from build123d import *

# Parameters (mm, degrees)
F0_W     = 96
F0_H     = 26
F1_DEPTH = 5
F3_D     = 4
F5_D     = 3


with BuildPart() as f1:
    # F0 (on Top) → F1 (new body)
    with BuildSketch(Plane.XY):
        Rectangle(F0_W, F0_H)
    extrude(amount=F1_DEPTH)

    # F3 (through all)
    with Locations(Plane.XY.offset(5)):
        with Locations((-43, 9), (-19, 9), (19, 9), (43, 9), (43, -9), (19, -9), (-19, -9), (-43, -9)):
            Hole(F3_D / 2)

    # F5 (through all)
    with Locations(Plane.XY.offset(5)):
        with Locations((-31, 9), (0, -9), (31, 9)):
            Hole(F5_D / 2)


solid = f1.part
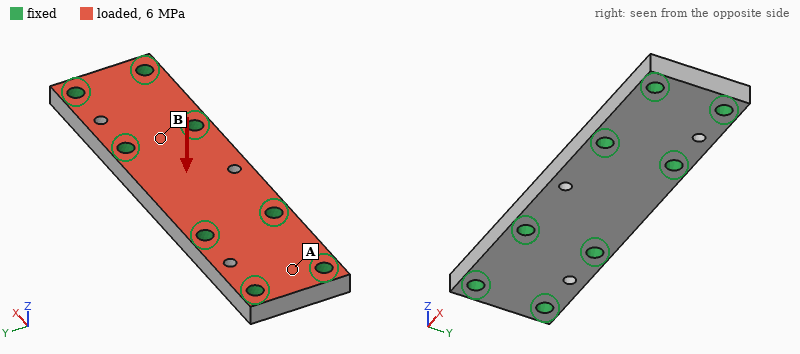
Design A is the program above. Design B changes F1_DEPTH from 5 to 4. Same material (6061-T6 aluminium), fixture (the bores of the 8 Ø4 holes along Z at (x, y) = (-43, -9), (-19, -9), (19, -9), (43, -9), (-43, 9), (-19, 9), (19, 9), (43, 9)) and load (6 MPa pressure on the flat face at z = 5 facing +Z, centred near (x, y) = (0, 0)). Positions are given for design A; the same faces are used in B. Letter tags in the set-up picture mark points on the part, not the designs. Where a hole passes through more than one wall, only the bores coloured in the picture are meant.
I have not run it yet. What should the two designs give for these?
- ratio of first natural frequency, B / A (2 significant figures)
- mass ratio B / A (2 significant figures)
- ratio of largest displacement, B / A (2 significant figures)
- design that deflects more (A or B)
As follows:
0.84
0.80
1.8
B
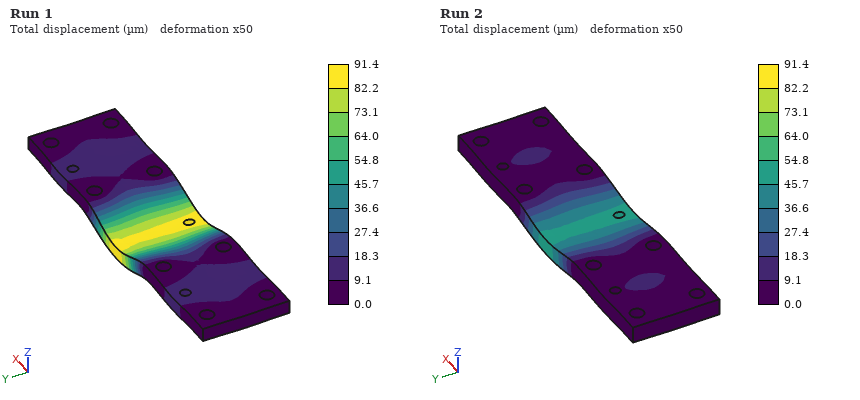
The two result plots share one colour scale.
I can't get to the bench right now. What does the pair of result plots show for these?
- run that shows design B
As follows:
Run 1
